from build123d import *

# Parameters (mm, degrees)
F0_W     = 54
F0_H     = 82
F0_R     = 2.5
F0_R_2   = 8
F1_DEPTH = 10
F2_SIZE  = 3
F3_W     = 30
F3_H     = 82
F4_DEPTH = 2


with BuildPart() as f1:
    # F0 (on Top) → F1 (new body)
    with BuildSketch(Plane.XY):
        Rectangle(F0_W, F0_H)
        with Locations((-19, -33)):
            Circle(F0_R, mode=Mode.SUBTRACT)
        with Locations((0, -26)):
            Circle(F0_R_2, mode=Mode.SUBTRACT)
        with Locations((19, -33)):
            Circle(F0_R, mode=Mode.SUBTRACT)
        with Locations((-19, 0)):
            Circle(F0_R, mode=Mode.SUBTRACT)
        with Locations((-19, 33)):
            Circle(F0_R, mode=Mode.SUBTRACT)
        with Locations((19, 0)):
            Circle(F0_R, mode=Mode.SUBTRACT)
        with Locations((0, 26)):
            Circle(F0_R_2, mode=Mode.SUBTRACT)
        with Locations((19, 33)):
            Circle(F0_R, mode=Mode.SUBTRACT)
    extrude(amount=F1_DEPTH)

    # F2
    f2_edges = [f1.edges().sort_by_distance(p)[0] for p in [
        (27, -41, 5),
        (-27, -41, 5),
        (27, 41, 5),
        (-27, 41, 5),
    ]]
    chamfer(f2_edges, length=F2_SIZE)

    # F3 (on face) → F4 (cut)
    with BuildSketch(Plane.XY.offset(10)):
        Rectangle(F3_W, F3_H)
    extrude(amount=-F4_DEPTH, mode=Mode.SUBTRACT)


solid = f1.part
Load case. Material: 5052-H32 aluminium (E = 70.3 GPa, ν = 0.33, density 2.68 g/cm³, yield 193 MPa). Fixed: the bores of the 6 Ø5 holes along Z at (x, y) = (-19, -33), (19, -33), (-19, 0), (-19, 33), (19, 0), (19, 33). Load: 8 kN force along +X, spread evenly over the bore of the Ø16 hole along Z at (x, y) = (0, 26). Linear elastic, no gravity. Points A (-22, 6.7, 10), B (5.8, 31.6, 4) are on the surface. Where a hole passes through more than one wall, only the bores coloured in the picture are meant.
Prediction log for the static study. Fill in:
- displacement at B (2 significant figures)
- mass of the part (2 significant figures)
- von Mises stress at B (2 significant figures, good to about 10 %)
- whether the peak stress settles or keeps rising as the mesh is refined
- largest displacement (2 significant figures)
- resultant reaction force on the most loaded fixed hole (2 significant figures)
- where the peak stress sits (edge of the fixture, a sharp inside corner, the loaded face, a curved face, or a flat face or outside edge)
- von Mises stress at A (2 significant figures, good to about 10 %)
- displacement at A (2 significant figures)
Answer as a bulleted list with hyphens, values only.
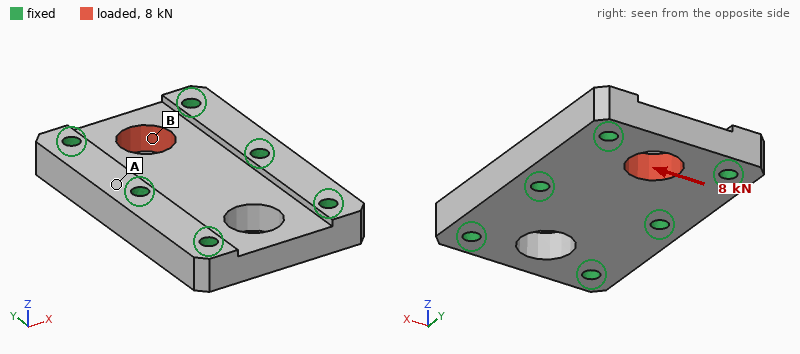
- 4.2 µm
- 93 g
- 30 MPa
- keeps rising
- 6.0 µm
- 2.9 kN
- edge of the fixture
- 7.0 MPa
- 1.5 µm
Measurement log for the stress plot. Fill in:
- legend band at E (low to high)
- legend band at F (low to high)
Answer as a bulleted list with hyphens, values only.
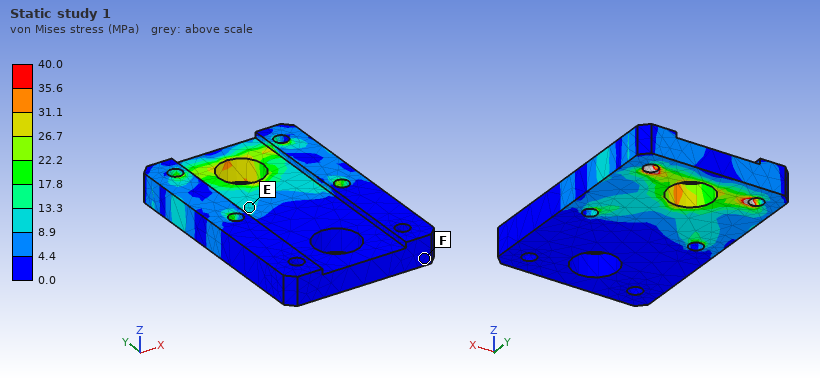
- 8.9 to 13.3 MPa
- 0.0 to 4.4 MPa
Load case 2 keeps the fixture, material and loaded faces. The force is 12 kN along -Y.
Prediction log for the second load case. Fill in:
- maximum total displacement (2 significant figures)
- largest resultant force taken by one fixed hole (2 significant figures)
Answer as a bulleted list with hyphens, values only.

- 23 µm
- 3.4 kN
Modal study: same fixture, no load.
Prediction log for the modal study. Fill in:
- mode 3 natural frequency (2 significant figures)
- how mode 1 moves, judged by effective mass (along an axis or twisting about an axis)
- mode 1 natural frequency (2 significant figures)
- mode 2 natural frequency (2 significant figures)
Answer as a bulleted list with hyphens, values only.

- 29 kHz
- along Z
- 22 kHz
- 25 kHz
